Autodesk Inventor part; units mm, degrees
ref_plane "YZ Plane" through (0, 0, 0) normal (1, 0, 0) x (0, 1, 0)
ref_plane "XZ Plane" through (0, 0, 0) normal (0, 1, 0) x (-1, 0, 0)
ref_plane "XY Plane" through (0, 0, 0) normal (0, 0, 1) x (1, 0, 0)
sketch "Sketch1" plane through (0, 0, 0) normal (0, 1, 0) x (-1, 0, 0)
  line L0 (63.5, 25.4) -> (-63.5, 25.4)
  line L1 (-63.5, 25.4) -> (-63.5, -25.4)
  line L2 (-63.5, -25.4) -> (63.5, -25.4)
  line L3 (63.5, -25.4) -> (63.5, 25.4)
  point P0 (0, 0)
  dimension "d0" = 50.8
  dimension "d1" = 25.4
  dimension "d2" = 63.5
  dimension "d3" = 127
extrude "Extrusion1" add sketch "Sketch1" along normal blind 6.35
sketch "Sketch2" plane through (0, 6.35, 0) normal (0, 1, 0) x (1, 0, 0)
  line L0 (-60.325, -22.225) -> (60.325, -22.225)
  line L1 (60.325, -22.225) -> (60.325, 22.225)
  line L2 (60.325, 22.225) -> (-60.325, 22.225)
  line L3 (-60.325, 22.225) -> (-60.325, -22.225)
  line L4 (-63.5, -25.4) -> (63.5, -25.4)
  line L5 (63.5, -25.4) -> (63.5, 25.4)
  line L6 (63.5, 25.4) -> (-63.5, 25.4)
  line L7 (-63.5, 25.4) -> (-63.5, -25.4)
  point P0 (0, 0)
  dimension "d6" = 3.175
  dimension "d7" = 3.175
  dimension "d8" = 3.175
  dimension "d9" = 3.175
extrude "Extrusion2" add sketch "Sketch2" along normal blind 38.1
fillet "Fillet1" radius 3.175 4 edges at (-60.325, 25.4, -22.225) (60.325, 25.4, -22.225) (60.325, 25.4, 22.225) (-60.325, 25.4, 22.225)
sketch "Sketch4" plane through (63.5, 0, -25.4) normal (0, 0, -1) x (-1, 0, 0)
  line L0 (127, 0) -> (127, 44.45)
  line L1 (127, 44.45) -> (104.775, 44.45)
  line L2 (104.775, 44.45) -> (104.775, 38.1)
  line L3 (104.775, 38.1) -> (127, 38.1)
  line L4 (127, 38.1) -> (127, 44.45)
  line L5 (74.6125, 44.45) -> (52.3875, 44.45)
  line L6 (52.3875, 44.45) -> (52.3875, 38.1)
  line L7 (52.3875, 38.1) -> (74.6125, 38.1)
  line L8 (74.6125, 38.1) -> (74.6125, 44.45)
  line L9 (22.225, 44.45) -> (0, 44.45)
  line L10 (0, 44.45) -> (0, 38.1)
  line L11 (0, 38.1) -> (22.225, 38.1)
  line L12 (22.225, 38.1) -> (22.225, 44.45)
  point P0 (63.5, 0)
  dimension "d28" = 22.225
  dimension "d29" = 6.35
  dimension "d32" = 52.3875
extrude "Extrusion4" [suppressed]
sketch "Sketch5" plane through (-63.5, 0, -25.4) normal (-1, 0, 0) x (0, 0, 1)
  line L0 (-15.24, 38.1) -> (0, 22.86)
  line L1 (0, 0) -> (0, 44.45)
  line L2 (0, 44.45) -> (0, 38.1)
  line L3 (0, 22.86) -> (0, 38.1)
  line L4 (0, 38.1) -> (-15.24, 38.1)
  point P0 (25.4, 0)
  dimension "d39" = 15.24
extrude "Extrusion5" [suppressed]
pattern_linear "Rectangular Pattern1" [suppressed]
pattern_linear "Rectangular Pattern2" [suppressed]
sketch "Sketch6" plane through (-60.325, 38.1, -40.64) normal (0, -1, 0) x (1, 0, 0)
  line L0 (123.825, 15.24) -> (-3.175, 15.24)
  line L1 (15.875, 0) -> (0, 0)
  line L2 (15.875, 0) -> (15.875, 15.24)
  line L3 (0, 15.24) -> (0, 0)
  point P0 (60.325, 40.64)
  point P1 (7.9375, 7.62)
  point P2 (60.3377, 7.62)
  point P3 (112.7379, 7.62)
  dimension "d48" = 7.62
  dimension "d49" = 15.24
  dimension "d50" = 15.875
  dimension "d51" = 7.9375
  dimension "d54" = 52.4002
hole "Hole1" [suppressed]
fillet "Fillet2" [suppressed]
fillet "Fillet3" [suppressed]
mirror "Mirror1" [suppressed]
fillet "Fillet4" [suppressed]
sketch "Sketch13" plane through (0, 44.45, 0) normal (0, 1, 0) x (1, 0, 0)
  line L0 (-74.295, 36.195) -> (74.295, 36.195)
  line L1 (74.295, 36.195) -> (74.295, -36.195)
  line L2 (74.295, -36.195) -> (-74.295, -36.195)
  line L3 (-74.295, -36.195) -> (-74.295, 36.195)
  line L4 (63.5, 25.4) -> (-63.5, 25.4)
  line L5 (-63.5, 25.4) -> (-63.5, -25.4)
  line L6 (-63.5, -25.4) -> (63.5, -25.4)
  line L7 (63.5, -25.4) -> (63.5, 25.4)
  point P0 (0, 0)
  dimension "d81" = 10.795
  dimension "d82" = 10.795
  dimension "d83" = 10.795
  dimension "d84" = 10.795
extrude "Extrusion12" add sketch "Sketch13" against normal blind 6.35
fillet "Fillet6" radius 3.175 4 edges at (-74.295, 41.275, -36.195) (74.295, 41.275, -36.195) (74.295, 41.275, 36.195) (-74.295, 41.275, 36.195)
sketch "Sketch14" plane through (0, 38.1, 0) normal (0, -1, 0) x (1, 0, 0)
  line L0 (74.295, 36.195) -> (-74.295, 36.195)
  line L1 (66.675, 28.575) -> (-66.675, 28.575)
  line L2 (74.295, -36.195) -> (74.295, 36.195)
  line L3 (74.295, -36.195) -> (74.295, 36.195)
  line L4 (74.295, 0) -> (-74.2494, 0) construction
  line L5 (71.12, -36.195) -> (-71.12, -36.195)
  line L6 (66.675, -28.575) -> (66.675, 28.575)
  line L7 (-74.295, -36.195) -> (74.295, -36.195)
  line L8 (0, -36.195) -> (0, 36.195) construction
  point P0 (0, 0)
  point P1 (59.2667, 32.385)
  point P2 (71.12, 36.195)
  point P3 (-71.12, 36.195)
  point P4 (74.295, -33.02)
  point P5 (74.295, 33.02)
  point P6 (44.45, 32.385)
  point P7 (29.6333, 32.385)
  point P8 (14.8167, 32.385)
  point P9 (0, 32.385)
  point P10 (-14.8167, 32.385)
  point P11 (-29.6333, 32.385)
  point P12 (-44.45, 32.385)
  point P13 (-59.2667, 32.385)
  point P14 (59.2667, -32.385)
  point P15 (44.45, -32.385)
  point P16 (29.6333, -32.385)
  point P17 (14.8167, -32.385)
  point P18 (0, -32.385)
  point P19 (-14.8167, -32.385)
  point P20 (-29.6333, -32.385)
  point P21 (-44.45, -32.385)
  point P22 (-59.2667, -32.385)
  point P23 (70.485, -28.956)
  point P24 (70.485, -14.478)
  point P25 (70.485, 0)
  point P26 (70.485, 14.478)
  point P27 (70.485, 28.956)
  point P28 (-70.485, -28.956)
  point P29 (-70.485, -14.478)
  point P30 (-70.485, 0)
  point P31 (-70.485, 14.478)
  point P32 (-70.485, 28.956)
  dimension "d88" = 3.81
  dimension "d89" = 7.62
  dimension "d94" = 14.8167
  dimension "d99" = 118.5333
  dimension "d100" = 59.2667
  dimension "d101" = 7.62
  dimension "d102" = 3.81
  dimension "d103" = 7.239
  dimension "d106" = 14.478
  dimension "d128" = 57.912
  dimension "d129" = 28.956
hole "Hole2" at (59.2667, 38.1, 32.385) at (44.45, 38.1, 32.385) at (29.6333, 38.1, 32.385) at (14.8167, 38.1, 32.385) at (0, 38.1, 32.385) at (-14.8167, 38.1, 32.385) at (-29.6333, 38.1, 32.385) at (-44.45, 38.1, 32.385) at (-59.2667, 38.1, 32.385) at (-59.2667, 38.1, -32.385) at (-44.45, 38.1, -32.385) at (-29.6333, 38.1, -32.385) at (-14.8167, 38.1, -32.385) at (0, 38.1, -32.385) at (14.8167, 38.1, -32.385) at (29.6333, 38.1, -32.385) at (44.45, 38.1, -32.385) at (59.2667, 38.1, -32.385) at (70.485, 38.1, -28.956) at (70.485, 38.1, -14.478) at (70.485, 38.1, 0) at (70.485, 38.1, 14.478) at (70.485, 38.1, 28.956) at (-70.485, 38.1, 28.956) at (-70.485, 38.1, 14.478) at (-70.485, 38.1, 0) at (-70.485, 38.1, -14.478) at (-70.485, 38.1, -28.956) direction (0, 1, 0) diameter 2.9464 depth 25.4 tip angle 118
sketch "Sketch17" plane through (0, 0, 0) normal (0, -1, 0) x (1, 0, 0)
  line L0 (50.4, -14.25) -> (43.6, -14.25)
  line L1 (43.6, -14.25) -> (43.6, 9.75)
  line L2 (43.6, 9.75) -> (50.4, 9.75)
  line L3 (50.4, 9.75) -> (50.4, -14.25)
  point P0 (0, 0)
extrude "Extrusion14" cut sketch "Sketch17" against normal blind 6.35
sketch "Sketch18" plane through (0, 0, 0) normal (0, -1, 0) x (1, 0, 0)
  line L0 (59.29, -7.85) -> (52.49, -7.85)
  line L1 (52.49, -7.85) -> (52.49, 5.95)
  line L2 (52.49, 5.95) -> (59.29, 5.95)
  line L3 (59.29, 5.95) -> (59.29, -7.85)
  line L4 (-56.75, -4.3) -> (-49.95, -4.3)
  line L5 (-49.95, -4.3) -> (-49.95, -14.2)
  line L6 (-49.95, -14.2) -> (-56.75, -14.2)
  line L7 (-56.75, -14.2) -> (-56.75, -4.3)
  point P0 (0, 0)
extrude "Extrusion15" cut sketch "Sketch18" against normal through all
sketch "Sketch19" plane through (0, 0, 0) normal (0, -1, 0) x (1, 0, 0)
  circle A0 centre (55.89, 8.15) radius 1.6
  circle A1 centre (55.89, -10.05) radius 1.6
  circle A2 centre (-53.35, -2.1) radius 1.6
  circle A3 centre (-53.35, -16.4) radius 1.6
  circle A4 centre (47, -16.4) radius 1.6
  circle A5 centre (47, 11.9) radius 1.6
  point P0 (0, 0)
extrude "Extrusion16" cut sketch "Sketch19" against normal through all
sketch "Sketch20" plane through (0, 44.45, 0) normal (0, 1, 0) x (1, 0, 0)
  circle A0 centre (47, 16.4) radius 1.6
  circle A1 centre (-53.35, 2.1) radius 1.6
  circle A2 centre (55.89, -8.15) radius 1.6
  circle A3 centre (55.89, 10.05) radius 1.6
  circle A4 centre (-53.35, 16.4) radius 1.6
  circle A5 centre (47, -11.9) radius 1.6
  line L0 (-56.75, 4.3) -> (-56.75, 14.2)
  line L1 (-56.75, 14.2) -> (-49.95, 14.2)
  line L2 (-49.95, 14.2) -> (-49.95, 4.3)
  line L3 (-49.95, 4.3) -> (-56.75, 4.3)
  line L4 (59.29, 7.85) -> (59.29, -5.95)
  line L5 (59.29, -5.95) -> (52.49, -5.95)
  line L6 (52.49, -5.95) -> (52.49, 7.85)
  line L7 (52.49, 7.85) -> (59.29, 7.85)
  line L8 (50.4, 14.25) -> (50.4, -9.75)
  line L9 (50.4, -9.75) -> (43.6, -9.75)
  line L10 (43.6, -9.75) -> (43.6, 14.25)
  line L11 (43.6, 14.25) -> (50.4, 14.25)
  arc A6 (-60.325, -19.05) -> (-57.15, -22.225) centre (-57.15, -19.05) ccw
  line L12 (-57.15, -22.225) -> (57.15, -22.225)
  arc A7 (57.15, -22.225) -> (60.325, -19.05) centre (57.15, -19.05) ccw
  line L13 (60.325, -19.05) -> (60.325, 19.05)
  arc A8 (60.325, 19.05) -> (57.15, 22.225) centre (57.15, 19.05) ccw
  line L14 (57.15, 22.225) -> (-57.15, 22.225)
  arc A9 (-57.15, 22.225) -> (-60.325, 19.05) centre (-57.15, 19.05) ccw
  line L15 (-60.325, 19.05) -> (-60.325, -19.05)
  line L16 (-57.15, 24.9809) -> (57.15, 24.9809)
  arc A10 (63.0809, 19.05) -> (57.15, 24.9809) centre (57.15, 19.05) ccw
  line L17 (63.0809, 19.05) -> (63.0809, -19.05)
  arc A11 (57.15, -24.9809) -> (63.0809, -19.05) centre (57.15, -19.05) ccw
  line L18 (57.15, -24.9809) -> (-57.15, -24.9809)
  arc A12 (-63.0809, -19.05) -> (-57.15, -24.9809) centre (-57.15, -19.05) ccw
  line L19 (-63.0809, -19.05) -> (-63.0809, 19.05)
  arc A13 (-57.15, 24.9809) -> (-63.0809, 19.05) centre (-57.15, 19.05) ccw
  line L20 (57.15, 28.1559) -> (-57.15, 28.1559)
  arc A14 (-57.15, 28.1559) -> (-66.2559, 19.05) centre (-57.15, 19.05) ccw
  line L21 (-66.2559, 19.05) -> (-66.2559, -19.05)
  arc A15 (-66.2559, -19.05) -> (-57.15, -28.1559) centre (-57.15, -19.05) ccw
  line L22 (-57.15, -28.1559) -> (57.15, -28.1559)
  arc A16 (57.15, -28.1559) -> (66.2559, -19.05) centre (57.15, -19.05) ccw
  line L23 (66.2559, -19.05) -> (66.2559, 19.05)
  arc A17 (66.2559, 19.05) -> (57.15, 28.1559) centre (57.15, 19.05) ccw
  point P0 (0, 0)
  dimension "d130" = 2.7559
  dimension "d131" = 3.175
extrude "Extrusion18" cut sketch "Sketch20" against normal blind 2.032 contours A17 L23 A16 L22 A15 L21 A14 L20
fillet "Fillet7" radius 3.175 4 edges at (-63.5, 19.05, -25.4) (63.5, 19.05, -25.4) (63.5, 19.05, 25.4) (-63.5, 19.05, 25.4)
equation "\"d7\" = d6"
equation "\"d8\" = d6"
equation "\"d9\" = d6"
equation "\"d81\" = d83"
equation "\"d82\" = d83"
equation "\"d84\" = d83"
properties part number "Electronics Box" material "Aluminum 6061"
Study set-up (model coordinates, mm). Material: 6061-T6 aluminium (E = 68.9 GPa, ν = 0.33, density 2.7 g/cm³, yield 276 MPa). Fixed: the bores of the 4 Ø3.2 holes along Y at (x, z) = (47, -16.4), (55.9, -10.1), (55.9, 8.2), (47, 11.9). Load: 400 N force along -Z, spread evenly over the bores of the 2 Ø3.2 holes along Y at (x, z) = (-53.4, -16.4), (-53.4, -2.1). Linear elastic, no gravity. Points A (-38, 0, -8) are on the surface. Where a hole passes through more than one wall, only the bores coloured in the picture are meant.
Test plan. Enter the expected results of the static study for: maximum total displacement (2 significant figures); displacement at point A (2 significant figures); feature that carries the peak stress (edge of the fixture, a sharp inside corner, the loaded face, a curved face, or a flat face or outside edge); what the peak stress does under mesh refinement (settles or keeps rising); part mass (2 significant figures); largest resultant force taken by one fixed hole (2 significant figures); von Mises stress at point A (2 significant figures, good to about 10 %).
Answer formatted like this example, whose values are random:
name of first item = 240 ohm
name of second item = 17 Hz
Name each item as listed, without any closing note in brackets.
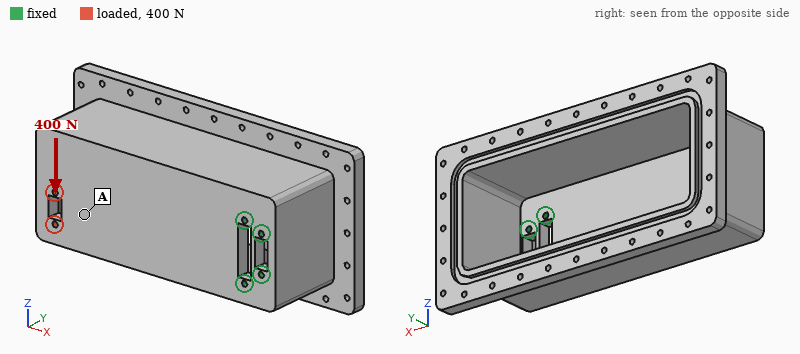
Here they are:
maximum total displacement = 48 µm
displacement at point A = 30 µm
feature that carries the peak stress = edge of the fixture
what the peak stress does under mesh refinement = keeps rising
part mass = 280 g
largest resultant force taken by one fixed hole = 1.2 kN
von Mises stress at point A = 2.4 MPa
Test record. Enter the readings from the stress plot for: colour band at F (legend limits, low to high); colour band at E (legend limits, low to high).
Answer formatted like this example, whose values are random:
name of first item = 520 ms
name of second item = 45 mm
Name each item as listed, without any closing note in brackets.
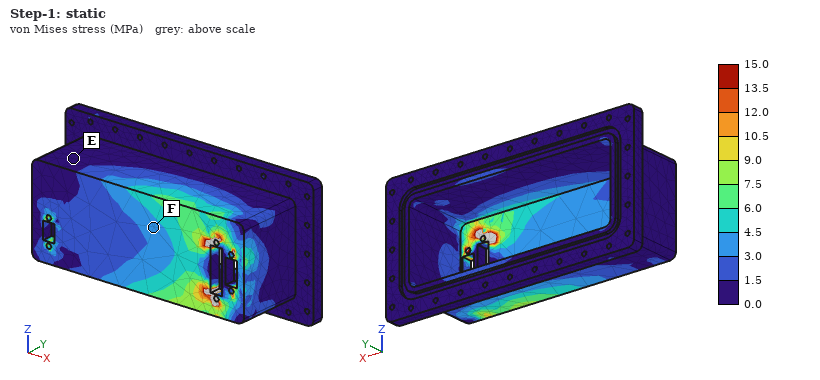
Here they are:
colour band at F = 3.0 to 4.5 MPa
colour band at E = 0.0 to 1.5 MPa
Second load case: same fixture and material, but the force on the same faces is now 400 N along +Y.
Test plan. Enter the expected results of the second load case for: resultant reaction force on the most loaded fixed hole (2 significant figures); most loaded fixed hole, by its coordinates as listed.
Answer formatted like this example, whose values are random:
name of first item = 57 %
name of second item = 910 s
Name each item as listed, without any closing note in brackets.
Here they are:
resultant reaction force on the most loaded fixed hole = 1.3 kN
most loaded fixed hole, by its coordinates as listed = (47, -16.4)
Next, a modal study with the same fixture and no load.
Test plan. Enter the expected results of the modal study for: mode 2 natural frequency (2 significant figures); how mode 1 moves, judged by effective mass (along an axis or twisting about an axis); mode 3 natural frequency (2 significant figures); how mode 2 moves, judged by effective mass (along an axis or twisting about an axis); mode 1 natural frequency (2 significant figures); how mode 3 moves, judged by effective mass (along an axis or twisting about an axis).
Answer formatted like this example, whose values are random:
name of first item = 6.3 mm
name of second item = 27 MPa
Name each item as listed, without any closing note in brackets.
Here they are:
mode 2 natural frequency = 970 Hz
how mode 1 moves, judged by effective mass = along Y
mode 3 natural frequency = 2000 Hz
how mode 2 moves, judged by effective mass = along Z
mode 1 natural frequency = 600 Hz
how mode 3 moves, judged by effective mass = along Z
